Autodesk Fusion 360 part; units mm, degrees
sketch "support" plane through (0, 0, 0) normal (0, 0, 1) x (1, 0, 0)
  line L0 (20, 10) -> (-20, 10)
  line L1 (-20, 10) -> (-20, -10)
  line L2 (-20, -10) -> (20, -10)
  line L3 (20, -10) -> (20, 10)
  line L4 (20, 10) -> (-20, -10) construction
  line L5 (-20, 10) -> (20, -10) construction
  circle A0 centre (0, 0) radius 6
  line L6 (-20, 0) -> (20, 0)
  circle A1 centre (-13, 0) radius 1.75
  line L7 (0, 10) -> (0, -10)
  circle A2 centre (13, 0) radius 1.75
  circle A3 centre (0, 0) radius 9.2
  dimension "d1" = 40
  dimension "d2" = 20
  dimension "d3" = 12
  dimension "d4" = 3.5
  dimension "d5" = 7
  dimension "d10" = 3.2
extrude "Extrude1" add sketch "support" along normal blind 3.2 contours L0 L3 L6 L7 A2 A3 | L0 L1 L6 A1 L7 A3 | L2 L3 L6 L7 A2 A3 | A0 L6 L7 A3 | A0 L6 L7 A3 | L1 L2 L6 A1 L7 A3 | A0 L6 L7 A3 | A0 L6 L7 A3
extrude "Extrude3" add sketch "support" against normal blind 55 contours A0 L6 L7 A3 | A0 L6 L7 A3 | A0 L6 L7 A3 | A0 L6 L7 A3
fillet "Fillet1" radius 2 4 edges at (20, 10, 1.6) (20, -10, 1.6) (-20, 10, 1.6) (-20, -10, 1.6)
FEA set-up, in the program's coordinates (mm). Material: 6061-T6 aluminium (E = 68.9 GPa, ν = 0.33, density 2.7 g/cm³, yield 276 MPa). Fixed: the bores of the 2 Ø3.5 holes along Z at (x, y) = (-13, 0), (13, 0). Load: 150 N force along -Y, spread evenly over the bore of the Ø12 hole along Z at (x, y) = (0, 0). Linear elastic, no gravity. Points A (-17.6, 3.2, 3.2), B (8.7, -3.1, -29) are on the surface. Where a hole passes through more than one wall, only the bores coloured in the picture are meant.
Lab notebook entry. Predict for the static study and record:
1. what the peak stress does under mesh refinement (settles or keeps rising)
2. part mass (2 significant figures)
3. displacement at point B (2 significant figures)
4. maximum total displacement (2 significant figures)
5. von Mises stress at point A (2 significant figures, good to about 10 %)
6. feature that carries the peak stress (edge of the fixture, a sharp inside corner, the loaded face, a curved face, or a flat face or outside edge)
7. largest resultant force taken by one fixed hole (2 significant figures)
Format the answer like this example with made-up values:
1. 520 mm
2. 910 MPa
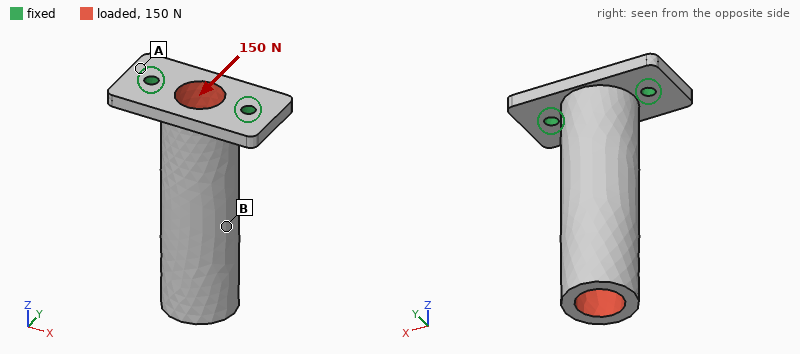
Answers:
1. keeps rising
2. 28 g
3. 0.068 mm
4. 0.13 mm
5. 17 MPa
6. edge of the fixture
7. 75 N
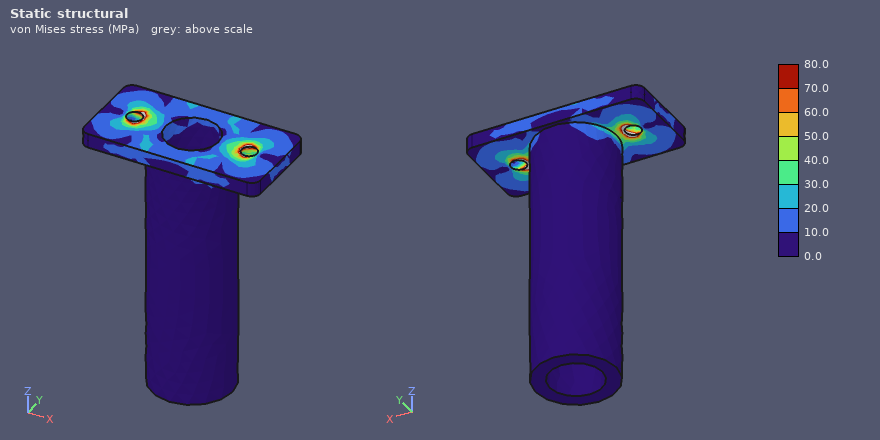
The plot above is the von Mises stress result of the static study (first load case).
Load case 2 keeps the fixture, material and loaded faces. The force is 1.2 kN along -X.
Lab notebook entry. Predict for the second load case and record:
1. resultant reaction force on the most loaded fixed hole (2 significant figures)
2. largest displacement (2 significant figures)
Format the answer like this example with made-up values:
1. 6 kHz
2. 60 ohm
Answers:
1. 1.7 kN
2. 0.19 mm
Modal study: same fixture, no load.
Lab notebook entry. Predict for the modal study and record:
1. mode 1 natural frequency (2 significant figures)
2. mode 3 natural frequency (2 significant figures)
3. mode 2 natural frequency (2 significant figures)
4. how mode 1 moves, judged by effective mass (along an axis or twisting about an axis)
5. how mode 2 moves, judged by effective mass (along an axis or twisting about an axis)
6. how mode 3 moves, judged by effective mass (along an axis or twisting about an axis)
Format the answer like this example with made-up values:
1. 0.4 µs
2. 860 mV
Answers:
1. 1300 Hz
2. 11 kHz
3. 3200 Hz
4. along Y
5. along X
6. along Z
